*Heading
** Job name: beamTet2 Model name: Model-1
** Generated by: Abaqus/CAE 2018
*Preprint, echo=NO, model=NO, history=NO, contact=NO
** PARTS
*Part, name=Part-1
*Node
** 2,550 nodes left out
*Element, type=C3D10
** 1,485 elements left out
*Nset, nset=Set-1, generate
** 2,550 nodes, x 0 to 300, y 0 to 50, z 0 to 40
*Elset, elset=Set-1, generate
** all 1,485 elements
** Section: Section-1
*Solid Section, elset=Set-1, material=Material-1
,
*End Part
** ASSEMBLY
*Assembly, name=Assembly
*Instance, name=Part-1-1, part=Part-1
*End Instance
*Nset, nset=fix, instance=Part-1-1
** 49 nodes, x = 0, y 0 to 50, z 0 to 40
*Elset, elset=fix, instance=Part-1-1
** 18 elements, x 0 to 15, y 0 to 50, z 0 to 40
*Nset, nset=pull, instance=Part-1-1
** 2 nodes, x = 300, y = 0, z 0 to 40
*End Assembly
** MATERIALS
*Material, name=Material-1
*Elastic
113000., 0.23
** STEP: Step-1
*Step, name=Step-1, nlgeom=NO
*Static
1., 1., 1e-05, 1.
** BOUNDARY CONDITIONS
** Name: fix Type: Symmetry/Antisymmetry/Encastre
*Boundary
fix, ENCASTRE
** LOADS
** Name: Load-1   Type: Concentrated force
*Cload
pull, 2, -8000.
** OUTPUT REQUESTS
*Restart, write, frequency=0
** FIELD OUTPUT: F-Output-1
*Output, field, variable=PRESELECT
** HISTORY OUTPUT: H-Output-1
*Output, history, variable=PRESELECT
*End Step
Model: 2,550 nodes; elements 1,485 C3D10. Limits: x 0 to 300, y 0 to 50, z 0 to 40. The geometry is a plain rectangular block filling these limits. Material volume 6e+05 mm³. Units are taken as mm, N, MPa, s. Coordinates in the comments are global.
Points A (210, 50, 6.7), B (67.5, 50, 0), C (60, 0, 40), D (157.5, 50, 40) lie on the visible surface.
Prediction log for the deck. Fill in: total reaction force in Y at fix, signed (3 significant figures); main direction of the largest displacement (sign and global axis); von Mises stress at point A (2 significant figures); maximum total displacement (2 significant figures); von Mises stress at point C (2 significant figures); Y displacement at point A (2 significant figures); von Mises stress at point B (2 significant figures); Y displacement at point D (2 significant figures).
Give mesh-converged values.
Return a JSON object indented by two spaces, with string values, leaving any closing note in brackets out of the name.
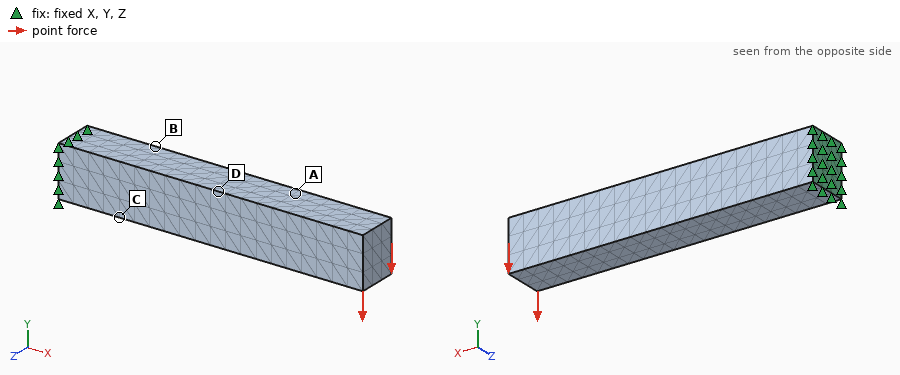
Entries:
{
  "total reaction force in Y at fix, signed": "16000 N",
  "main direction of the largest displacement": "-Y",
  "von Mises stress at point A": "86 MPa",
  "maximum total displacement": "3.2 mm",
  "von Mises stress at point C": "230 MPa",
  "Y displacement at point A": "-1.8 mm",
  "von Mises stress at point B": "220 MPa",
  "Y displacement at point D": "-1.1 mm"
}
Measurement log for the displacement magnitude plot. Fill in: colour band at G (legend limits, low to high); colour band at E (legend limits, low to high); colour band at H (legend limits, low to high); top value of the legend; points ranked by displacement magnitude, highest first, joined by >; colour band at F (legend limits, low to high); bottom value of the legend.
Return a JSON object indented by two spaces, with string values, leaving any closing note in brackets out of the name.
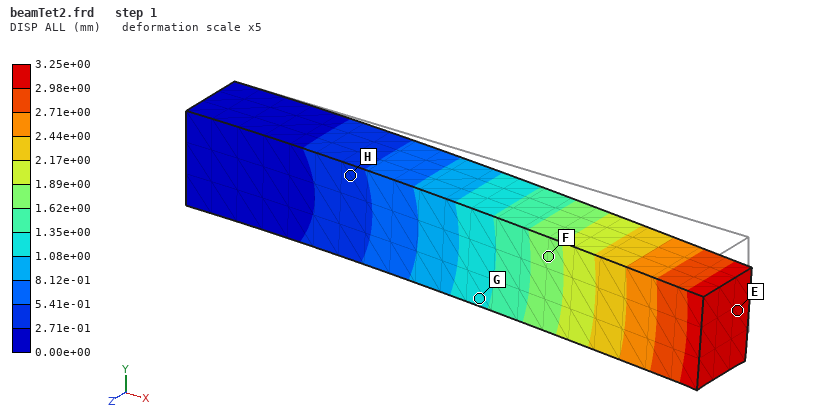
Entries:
{
  "colour band at G": "1.08e+00 to 1.35e+00 mm",
  "colour band at E": "2.98e+00 to 3.25e+00 mm",
  "colour band at H": "2.71e-01 to 5.41e-01 mm",
  "top value of the legend": "3.25e+00 mm",
  "points ranked by displacement magnitude, highest first, joined by >": "E > F > G > H",
  "colour band at F": "1.62e+00 to 1.89e+00 mm",
  "bottom value of the legend": "0.00e+00 mm"
}
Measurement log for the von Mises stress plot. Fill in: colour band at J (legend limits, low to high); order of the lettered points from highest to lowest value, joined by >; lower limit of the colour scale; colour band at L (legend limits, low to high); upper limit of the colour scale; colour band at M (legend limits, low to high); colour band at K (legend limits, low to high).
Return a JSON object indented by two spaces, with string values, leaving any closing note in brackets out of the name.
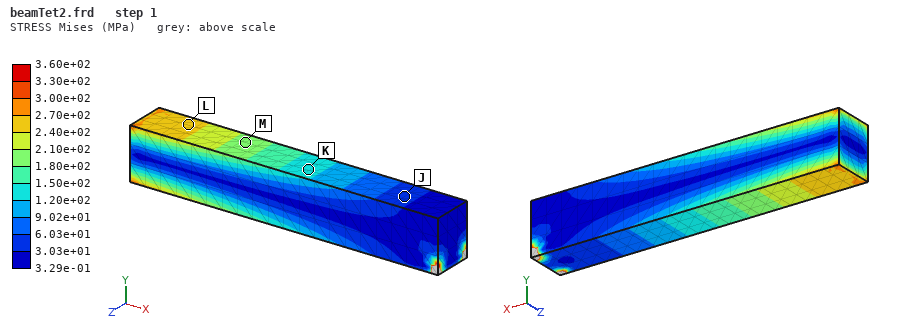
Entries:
{
  "colour band at J": "3.03e+01 to 6.03e+01 MPa",
  "order of the lettered points from highest to lowest value, joined by >": "L > M > K > J",
  "lower limit of the colour scale": "3.29e-01 MPa",
  "colour band at L": "2.40e+02 to 2.70e+02 MPa",
  "upper limit of the colour scale": "3.60e+02 MPa",
  "colour band at M": "1.80e+02 to 2.10e+02 MPa",
  "colour band at K": "1.20e+02 to 1.50e+02 MPa"
}
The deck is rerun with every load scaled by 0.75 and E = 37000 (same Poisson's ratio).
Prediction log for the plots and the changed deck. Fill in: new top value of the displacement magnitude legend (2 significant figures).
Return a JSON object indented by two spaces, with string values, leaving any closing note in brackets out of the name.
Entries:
{
  "new top value of the displacement magnitude legend": "7.4 mm"
}
